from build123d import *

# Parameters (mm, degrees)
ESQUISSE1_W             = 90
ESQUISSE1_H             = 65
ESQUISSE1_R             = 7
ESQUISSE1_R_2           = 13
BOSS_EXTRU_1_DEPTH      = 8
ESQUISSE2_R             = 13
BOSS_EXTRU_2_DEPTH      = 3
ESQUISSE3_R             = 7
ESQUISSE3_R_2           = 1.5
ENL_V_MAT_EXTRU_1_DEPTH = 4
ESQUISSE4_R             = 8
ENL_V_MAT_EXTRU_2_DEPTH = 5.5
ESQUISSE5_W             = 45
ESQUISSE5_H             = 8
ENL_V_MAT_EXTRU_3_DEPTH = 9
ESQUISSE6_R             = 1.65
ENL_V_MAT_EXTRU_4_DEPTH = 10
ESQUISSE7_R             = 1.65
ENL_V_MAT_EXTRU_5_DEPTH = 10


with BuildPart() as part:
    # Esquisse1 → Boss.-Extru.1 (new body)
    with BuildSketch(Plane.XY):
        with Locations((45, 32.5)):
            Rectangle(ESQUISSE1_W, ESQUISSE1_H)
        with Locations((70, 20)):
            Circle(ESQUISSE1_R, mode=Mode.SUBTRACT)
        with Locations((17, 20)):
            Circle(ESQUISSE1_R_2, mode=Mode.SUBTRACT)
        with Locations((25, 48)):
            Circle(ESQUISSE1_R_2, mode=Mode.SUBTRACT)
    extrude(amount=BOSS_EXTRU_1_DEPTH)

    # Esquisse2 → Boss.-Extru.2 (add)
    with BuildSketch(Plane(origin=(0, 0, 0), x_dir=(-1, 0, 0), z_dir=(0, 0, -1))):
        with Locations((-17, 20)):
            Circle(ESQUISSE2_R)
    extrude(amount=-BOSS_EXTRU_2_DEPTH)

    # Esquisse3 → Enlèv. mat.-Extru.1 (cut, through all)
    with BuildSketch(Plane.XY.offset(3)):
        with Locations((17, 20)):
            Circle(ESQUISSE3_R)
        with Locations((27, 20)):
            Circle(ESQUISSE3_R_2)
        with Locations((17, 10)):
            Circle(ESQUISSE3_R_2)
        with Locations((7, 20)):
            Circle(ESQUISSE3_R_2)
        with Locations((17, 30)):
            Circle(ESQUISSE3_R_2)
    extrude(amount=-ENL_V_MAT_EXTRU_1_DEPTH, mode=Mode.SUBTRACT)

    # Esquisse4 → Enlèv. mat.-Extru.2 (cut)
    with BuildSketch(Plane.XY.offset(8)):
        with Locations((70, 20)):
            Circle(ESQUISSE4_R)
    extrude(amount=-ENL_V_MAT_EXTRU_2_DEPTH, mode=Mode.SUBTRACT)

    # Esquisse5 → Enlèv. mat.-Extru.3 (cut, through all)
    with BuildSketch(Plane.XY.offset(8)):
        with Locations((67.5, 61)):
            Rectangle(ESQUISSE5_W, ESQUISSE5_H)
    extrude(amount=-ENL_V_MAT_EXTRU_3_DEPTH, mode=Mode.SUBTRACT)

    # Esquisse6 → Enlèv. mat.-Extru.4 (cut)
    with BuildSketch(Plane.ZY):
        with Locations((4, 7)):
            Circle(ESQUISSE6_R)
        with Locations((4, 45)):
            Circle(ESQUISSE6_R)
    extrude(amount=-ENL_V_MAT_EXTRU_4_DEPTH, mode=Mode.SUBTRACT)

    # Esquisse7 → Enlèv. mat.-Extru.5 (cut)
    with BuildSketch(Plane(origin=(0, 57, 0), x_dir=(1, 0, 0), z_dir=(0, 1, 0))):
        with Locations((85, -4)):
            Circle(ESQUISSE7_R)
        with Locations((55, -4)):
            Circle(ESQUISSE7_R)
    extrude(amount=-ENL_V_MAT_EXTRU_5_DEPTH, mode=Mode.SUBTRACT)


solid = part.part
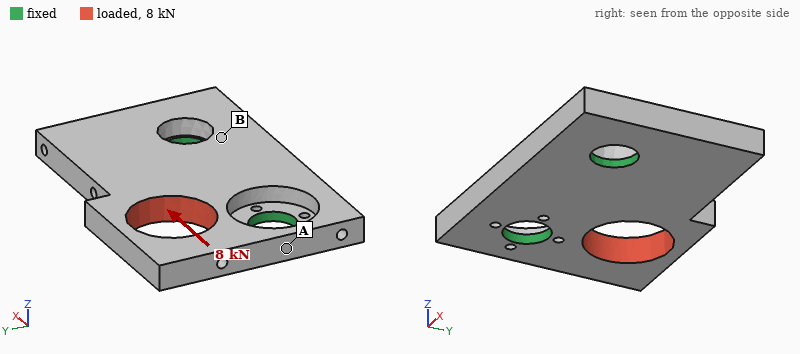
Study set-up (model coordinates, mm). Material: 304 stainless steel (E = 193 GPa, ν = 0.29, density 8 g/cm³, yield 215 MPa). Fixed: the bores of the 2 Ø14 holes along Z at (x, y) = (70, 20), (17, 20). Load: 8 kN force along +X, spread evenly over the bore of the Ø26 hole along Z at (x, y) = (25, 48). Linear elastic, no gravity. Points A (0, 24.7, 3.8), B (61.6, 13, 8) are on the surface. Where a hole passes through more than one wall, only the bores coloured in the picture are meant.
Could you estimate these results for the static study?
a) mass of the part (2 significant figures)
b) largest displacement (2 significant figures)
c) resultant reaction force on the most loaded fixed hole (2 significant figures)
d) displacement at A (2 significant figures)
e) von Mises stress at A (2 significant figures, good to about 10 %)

280 g
28 µm
5.2 kN
7.3 µm
48 MPa
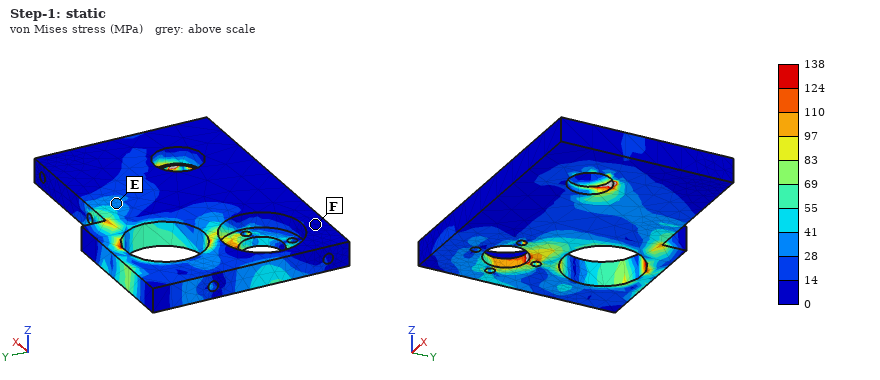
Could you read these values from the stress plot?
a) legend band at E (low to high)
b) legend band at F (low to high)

28 to 41 MPa
0 to 14 MPa
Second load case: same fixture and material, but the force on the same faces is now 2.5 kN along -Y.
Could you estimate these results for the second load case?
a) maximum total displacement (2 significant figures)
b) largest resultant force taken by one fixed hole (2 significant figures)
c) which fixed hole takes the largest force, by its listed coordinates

16 µm
2.0 kN
(17, 20)
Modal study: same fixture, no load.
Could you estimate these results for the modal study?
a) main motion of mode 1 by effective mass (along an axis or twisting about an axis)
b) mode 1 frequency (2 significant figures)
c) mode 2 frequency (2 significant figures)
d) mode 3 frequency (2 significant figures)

along Z
2500 Hz
4100 Hz
6700 Hz
